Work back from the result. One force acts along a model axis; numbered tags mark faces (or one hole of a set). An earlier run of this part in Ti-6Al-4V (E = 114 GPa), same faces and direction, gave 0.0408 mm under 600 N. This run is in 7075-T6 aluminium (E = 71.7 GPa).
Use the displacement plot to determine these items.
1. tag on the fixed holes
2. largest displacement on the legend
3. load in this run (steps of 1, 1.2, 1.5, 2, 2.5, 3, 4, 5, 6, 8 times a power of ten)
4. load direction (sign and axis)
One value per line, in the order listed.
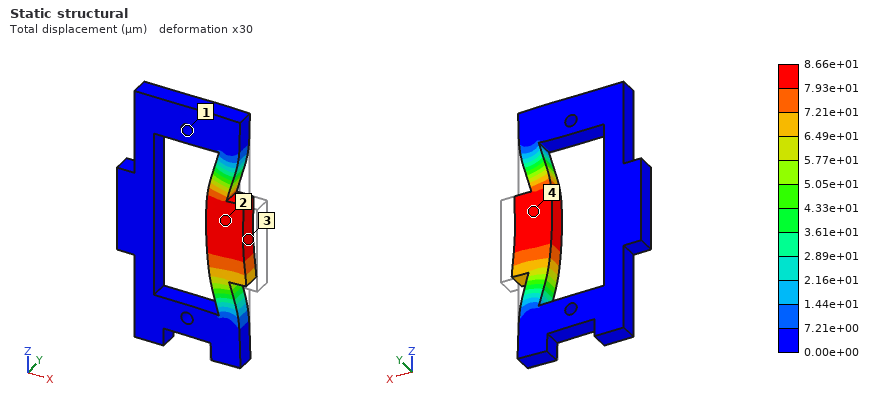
1
8.66e+01 µm
800 N
-X
